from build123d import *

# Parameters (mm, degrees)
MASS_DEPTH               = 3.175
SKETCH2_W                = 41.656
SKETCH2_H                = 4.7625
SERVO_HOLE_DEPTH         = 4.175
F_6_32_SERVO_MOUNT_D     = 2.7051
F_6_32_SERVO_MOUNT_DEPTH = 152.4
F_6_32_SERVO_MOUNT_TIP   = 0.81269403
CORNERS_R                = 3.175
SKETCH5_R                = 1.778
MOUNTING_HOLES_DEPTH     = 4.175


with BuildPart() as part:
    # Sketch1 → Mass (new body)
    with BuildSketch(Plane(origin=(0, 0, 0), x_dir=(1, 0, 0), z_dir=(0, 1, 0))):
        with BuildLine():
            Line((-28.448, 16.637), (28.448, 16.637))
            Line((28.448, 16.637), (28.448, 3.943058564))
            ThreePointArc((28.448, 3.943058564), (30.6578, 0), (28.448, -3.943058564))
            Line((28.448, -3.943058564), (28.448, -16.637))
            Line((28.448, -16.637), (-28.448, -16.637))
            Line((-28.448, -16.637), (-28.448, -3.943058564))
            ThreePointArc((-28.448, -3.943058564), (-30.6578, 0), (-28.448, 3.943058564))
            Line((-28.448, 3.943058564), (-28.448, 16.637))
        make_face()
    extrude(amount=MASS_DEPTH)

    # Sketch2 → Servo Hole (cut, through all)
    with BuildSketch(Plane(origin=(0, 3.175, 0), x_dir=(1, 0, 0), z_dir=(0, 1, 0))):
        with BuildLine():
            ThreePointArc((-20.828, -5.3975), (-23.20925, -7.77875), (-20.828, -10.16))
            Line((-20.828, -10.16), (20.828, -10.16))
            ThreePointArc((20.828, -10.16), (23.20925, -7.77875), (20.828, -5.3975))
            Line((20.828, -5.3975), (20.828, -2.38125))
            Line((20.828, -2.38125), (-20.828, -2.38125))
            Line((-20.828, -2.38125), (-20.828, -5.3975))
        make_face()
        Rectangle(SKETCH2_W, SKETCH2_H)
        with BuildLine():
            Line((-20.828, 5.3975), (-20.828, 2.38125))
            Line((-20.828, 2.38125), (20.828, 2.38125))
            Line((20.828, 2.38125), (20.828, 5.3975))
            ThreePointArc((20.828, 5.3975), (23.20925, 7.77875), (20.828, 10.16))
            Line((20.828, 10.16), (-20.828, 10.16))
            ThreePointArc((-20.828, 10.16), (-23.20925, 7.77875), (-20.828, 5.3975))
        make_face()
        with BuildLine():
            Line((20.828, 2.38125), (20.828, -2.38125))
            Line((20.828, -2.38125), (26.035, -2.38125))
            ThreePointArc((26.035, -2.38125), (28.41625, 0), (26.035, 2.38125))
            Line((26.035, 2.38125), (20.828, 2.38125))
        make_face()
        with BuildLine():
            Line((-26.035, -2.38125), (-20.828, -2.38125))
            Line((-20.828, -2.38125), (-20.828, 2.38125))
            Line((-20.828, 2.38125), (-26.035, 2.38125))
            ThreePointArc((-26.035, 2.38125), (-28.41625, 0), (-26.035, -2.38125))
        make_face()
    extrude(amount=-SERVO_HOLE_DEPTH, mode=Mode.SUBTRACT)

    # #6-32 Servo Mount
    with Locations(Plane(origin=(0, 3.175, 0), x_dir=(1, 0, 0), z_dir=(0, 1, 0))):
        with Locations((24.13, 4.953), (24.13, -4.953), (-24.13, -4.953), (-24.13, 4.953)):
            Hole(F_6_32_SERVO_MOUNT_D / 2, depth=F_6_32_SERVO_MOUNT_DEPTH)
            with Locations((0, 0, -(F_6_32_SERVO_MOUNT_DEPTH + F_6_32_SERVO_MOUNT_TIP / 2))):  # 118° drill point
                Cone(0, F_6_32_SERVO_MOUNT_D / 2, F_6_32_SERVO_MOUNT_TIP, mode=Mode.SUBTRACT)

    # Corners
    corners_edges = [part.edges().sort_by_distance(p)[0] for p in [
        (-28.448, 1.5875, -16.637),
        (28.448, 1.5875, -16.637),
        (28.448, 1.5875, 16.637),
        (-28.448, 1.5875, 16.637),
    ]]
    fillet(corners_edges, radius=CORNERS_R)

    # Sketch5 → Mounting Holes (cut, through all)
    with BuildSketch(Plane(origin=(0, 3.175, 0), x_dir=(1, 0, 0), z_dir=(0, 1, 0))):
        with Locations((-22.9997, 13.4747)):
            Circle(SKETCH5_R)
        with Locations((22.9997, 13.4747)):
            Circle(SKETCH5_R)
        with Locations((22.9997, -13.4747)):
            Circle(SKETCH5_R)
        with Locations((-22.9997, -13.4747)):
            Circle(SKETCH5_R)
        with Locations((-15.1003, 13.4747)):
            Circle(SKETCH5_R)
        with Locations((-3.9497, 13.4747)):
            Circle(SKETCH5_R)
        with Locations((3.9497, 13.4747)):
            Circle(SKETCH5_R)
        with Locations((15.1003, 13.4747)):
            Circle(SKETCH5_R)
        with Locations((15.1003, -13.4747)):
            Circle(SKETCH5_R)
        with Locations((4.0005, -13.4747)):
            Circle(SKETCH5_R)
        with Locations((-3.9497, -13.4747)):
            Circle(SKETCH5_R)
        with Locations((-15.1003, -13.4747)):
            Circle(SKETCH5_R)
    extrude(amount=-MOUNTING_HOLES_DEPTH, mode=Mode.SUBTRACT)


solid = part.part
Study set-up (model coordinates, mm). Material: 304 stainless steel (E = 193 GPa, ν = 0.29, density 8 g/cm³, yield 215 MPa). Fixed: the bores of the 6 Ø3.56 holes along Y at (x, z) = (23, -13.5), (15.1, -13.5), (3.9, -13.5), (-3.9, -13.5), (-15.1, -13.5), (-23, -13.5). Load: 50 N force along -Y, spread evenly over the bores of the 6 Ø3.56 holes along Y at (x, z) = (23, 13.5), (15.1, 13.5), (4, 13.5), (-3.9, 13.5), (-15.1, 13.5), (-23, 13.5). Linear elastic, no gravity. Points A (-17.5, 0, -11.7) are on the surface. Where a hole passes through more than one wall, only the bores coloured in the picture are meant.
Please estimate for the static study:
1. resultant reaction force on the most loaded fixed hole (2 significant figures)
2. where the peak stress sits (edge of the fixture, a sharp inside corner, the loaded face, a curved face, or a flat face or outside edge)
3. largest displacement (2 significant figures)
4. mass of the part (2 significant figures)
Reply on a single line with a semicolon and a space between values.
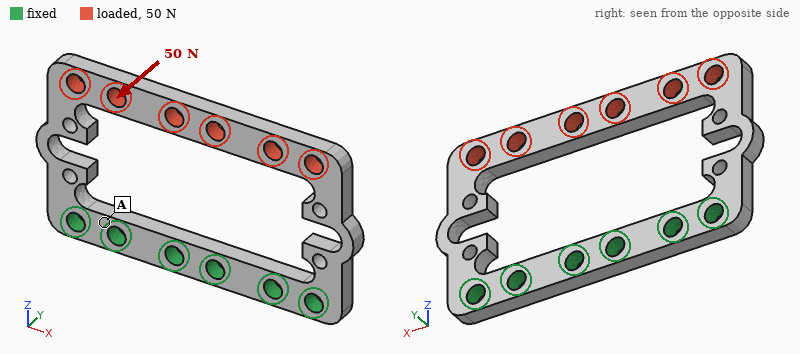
30 N; a flat face or outside edge; 0.15 mm; 21 g
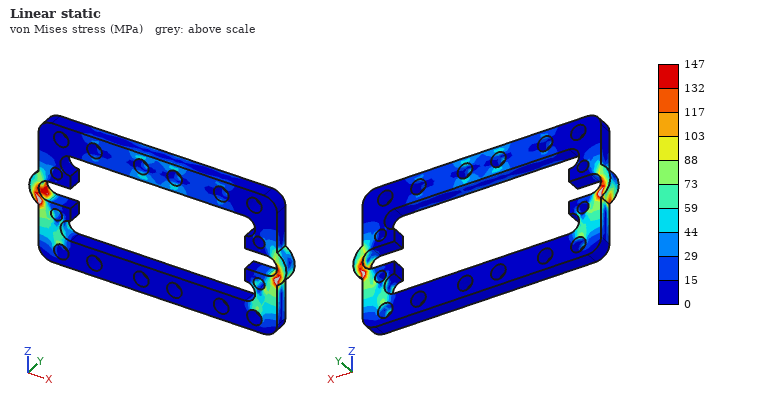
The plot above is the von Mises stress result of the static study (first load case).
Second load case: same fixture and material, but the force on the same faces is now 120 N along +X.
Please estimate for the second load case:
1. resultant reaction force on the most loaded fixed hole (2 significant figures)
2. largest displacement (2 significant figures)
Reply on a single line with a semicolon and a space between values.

64 N; 26 µm
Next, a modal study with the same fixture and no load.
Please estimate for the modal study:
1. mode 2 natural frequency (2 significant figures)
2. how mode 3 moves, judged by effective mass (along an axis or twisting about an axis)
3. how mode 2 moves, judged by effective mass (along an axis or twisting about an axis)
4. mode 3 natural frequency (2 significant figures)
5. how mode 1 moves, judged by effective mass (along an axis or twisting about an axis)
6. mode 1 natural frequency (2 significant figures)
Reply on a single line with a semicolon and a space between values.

2800 Hz; along X; twisting about Z; 3600 Hz; along Y; 1100 Hz
